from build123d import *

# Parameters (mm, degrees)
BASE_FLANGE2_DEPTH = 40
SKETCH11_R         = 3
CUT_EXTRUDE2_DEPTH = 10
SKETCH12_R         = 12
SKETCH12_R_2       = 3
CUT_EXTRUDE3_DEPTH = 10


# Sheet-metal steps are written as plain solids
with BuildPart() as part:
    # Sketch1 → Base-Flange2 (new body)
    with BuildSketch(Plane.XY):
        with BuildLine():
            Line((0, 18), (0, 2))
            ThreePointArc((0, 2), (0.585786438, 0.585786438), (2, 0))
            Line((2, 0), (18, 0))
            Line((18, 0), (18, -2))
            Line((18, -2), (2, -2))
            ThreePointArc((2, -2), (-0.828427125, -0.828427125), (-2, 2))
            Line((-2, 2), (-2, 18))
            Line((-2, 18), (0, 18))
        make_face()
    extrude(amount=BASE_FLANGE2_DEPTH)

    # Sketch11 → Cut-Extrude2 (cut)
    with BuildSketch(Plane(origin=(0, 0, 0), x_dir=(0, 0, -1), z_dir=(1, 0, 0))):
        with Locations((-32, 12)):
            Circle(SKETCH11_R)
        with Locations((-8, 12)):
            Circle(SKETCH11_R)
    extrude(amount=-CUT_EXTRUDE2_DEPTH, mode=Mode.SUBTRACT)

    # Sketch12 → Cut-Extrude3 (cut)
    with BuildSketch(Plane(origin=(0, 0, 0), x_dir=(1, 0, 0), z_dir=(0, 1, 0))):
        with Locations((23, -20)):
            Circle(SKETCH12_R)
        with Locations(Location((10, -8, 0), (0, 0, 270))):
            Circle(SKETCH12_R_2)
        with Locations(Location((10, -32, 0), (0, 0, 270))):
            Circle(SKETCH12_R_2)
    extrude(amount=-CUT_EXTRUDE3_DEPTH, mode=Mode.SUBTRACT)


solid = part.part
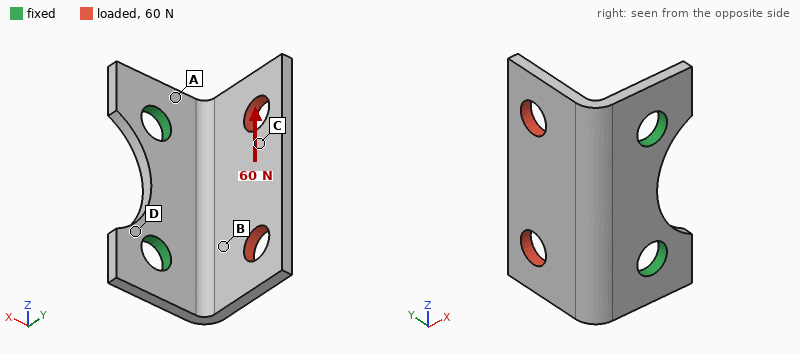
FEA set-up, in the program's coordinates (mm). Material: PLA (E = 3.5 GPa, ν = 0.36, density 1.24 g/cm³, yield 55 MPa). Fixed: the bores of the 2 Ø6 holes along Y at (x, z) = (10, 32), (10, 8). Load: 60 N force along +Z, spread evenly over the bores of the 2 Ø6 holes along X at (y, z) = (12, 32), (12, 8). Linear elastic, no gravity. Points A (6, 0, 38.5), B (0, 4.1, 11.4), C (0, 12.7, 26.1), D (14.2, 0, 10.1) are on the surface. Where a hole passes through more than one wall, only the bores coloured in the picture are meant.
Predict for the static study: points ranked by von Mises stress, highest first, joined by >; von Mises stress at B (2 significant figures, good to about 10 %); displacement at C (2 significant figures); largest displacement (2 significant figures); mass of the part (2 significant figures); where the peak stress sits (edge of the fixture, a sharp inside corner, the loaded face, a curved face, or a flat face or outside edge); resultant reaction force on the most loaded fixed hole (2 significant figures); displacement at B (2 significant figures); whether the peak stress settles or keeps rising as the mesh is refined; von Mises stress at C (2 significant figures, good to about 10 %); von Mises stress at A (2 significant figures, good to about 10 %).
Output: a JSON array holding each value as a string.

["A > B > C > D", "5.9 MPa", "0.16 mm", "0.34 mm", "3.1 g", "edge of the fixture", "46 N", "0.097 mm", "keeps rising", "3.3 MPa", "9.0 MPa"]
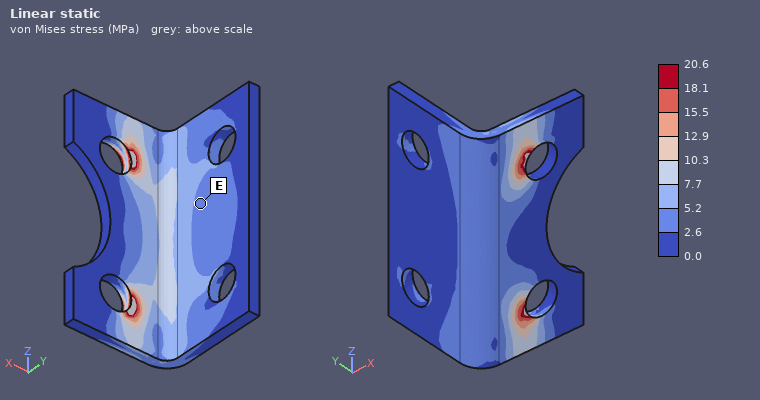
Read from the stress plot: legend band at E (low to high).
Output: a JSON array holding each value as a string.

["2.6 to 5.2 MPa"]
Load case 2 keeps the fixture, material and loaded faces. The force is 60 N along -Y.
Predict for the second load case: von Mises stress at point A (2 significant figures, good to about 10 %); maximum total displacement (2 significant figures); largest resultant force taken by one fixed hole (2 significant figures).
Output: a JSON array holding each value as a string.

["12 MPa", "0.56 mm", "30 N"]
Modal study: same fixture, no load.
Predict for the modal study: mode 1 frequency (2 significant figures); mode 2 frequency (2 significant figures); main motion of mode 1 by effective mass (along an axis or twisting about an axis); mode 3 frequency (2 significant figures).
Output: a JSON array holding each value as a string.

["940 Hz", "1600 Hz", "along X", "2900 Hz"]
